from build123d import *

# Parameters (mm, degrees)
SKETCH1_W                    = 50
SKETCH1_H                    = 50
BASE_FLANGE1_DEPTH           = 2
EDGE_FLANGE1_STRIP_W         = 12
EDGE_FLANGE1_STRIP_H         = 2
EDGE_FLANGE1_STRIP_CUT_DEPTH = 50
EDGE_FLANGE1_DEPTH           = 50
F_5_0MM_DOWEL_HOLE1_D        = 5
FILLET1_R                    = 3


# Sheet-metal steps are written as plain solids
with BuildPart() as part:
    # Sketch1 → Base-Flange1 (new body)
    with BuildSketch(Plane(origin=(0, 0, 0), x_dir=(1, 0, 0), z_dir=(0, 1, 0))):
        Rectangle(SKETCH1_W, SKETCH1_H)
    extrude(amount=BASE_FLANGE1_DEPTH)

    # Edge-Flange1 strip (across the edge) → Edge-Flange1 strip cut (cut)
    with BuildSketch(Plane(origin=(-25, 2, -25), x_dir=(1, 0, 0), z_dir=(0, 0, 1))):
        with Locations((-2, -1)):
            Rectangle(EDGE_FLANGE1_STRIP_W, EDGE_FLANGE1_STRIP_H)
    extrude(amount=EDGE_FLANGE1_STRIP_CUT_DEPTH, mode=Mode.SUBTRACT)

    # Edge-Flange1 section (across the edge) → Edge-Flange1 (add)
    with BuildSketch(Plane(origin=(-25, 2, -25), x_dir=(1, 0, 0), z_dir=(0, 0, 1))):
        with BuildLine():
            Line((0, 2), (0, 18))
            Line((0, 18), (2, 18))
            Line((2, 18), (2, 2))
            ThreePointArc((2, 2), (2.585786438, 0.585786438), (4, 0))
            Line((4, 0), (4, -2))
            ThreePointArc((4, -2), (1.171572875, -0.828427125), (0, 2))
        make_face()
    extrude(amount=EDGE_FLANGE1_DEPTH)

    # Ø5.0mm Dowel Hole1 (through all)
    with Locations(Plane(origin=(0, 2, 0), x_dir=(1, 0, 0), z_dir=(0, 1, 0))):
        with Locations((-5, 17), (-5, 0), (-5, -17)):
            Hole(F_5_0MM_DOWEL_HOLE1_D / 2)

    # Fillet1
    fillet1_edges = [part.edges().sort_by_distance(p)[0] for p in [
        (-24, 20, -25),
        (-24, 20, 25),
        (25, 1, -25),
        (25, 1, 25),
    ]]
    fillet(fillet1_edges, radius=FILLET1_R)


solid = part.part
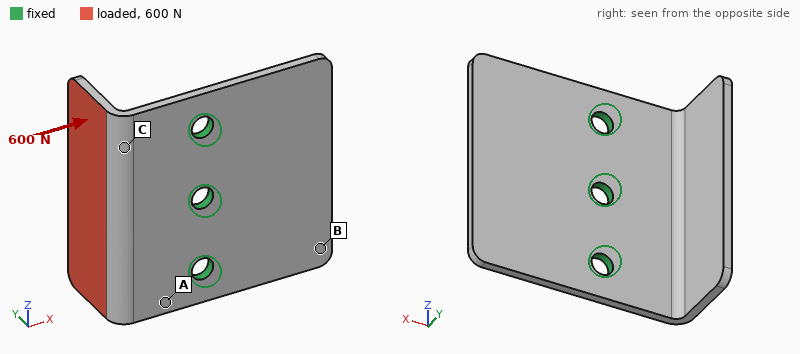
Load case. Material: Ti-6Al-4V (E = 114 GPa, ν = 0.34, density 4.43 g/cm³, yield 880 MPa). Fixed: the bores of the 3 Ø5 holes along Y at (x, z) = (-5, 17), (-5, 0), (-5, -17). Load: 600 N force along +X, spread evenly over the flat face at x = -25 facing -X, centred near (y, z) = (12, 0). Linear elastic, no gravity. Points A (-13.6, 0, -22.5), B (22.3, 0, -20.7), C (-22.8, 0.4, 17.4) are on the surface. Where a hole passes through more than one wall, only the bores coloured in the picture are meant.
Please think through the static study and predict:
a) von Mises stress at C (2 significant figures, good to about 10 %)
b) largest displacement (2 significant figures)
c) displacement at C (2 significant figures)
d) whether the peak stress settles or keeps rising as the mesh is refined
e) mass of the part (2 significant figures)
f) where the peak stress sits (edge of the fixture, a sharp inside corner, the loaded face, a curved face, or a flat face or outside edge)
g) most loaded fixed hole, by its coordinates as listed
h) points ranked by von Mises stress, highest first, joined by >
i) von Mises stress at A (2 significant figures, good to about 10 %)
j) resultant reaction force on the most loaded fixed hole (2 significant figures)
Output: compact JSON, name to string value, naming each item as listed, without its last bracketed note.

{"von Mises stress at C": "140 MPa", "largest displacement": "0.69 mm", "displacement at C": "0.22 mm", "whether the peak stress settles or keeps rising as the mesh is refined": "keeps rising", "mass of the part": "29 g", "where the peak stress sits": "edge of the fixture", "most loaded fixed hole, by its coordinates as listed": "(-5, 0)", "points ranked by von Mises stress, highest first, joined by >": "A > C > B", "von Mises stress at A": "190 MPa", "resultant reaction force on the most loaded fixed hole": "220 N"}
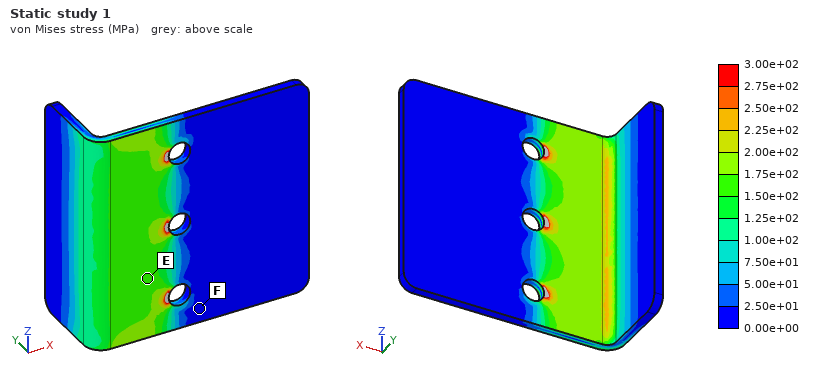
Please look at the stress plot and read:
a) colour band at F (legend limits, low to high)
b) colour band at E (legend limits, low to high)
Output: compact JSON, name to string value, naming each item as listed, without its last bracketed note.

{"colour band at F": "0.00e+00 to 2.50e+01 MPa", "colour band at E": "1.50e+02 to 1.75e+02 MPa"}
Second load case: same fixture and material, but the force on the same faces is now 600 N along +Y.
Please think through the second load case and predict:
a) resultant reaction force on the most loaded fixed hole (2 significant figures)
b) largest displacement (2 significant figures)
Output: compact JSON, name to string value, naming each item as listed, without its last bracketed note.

{"resultant reaction force on the most loaded fixed hole": "210 N", "largest displacement": "0.59 mm"}
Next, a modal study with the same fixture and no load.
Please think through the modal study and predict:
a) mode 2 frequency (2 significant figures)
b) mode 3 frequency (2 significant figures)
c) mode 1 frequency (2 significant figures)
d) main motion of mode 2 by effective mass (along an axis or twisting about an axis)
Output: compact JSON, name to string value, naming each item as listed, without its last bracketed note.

{"mode 2 frequency": "2100 Hz", "mode 3 frequency": "2800 Hz", "mode 1 frequency": "1700 Hz", "main motion of mode 2 by effective mass": "along Y"}
